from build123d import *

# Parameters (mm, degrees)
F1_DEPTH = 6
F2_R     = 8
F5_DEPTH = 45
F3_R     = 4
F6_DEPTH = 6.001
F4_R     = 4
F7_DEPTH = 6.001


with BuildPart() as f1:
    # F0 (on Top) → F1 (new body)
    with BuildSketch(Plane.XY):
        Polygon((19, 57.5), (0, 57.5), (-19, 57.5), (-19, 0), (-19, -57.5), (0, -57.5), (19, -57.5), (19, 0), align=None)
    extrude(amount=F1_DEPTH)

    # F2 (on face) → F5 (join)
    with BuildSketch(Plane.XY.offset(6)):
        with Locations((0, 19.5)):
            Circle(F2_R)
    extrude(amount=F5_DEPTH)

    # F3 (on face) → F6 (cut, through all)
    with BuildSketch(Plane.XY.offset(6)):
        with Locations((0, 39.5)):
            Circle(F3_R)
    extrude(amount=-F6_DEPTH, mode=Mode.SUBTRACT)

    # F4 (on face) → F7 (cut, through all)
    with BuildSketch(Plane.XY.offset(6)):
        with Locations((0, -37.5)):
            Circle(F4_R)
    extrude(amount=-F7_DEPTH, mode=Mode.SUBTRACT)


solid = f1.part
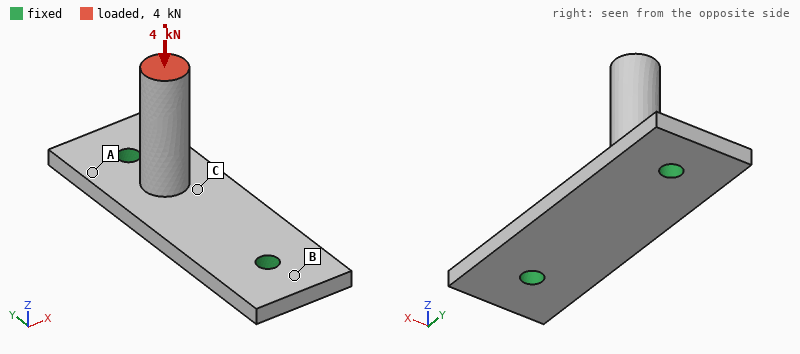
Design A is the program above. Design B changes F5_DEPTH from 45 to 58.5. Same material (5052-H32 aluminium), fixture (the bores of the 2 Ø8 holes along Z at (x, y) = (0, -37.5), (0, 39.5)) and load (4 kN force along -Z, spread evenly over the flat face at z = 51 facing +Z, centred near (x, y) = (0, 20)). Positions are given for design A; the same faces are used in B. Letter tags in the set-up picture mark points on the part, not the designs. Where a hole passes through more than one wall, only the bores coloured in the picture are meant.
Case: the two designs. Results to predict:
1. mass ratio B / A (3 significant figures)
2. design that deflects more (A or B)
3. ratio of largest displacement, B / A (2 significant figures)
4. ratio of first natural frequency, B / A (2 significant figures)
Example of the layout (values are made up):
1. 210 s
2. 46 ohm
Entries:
1. 1.08
2. B
3. 1.2
4. 0.69
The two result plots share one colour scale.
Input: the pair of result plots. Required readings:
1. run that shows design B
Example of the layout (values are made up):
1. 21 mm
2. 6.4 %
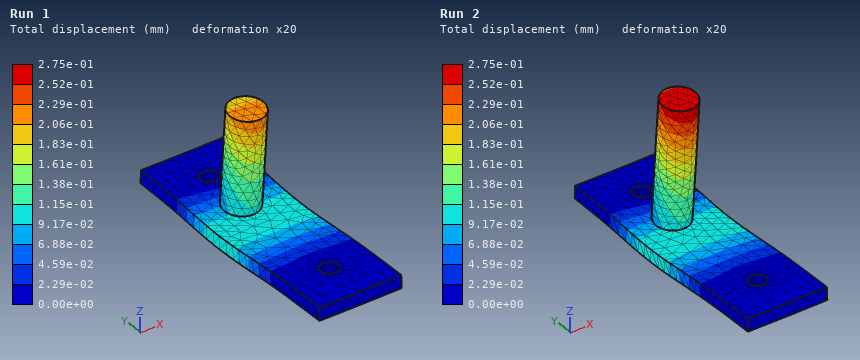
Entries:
1. Run 2
